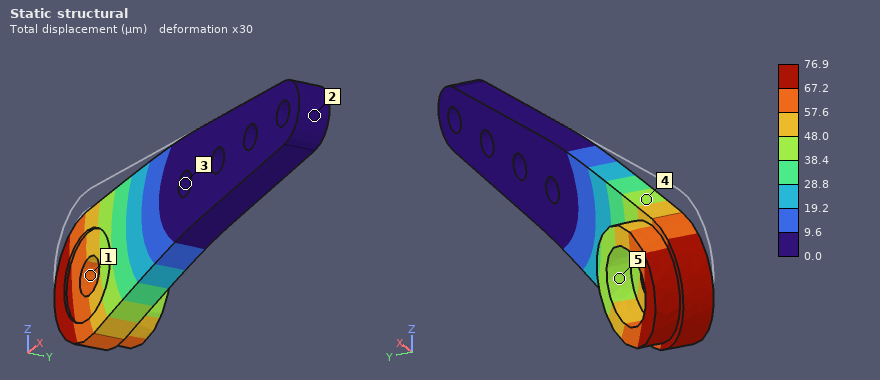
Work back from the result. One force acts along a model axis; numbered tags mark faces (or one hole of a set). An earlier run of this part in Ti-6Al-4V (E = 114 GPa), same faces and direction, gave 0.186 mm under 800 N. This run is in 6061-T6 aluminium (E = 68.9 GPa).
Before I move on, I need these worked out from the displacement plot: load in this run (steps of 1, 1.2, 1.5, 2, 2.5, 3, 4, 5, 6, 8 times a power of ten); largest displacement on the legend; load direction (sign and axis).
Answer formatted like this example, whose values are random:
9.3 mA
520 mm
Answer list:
200 N
76.9 µm
-Z
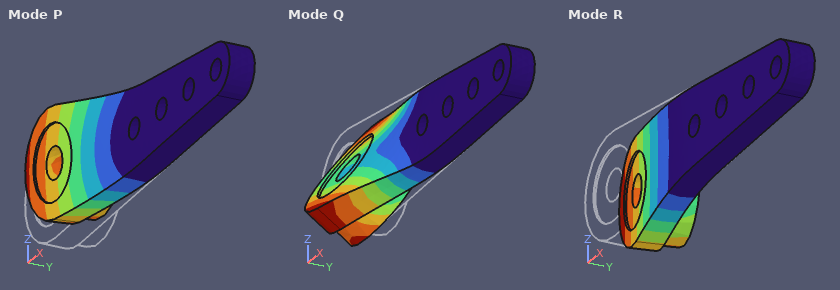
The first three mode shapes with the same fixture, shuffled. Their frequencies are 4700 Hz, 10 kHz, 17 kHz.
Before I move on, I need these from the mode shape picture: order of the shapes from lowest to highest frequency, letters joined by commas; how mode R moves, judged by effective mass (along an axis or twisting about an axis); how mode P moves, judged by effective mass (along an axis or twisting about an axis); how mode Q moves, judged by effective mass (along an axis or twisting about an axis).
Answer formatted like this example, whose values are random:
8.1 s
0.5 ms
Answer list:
R, P, Q
along Y
along Z
twisting about X
